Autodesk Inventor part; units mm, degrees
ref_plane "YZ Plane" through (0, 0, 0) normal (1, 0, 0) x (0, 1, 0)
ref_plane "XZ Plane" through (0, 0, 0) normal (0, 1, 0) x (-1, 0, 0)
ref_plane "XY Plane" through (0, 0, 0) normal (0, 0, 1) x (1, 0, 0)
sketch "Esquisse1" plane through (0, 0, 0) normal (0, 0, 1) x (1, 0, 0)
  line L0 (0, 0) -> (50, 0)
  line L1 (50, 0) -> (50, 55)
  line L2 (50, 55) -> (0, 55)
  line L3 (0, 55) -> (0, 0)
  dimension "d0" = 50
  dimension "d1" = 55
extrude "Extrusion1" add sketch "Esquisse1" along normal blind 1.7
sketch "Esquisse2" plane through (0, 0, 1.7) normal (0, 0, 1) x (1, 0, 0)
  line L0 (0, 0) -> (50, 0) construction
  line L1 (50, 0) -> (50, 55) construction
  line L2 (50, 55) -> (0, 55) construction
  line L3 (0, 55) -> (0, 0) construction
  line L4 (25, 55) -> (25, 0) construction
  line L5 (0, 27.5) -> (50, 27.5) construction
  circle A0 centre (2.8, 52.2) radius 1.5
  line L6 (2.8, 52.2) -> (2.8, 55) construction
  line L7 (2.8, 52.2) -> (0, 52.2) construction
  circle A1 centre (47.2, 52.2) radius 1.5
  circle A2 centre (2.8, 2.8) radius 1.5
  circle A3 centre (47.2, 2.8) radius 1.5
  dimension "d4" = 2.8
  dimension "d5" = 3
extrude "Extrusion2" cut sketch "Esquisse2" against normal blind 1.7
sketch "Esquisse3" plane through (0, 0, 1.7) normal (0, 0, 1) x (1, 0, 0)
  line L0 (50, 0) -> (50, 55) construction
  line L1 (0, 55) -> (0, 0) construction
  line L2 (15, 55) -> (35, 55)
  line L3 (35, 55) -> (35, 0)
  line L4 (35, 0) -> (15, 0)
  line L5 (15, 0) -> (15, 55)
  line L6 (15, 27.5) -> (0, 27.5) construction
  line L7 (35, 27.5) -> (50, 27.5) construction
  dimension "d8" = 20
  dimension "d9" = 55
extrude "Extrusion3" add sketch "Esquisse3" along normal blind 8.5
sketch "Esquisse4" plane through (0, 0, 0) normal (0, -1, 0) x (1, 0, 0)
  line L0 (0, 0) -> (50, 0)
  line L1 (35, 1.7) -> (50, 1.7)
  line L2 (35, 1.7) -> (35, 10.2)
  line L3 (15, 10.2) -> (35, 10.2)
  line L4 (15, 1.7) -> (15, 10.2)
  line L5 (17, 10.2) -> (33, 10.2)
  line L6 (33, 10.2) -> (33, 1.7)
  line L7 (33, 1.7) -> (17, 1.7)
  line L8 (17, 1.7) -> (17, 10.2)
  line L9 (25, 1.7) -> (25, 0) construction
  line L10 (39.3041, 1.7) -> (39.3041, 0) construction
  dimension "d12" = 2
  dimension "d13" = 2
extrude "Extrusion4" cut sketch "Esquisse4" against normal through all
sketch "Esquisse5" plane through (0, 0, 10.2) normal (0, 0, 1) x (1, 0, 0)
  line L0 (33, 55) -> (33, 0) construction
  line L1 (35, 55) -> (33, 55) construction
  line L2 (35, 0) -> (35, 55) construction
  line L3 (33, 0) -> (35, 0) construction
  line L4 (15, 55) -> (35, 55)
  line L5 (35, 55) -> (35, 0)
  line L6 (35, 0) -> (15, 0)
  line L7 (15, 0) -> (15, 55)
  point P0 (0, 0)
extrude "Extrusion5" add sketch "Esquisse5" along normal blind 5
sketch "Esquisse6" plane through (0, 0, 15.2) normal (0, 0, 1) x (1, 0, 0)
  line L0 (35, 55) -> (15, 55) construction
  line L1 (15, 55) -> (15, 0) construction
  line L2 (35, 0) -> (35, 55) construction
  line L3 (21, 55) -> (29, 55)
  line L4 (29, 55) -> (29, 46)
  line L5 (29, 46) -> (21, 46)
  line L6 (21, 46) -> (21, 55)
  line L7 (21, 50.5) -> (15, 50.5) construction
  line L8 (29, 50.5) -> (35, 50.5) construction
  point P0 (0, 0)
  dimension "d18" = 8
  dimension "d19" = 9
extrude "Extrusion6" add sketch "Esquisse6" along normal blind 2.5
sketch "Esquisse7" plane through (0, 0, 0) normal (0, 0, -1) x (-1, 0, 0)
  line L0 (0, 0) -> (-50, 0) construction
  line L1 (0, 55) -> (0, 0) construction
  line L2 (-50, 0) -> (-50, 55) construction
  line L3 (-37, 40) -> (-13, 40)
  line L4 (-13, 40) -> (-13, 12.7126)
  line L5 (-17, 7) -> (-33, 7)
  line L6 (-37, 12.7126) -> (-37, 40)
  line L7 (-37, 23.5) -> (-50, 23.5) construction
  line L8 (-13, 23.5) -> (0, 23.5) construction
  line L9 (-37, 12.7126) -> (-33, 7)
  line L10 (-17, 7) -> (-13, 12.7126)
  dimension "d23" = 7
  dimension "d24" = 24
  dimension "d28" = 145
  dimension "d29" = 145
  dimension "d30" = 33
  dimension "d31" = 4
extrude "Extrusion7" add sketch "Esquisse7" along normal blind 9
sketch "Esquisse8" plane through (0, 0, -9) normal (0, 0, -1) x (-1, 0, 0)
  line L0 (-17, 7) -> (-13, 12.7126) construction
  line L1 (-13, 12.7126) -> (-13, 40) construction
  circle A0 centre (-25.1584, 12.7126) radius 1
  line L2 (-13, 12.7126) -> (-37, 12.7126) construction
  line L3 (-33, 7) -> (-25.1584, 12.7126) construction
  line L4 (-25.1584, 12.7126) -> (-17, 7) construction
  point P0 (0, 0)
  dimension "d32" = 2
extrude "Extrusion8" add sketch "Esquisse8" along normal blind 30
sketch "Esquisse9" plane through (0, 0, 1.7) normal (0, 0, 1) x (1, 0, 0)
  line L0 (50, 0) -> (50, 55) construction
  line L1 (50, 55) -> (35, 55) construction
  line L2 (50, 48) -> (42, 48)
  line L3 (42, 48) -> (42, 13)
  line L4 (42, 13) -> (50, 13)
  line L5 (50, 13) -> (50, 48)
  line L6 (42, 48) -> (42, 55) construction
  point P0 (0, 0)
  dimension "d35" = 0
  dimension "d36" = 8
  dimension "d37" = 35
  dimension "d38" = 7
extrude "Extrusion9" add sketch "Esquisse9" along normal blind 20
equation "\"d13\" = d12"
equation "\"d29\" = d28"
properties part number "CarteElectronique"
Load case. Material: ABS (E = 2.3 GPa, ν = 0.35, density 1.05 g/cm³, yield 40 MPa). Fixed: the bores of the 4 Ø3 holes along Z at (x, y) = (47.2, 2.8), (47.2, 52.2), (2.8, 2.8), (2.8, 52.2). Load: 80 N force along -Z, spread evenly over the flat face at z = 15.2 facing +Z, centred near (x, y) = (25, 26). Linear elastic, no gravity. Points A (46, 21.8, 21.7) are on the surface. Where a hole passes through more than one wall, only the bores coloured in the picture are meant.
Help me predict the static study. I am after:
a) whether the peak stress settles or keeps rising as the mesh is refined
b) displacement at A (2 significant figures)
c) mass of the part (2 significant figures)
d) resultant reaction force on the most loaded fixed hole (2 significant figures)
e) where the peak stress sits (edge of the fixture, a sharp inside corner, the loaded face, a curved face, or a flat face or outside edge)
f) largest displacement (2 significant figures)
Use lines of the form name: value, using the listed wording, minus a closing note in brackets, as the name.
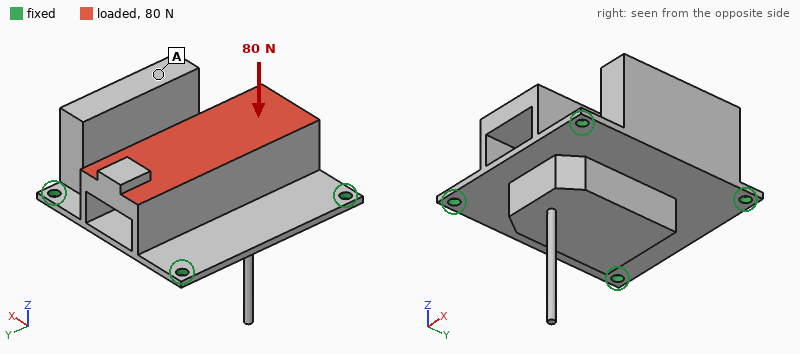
whether the peak stress settles or keeps rising as the mesh is refined: keeps rising
displacement at A: 0.36 mm
mass of the part: 26 g
resultant reaction force on the most loaded fixed hole: 23 N
where the peak stress sits: edge of the fixture
largest displacement: 0.39 mm
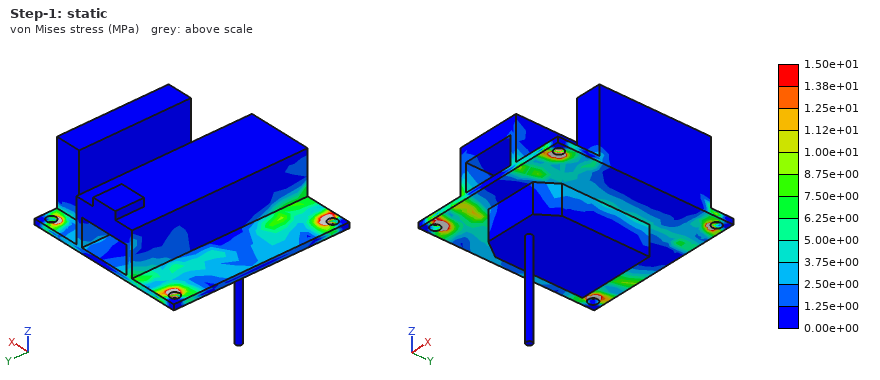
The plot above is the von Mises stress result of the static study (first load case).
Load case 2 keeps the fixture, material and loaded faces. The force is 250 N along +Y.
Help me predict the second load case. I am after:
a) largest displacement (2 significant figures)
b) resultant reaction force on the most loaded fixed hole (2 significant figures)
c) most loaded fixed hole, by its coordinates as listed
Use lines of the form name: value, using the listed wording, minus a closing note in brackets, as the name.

largest displacement: 0.76 mm
resultant reaction force on the most loaded fixed hole: 94 N
most loaded fixed hole, by its coordinates as listed: (47.2, 52.2)
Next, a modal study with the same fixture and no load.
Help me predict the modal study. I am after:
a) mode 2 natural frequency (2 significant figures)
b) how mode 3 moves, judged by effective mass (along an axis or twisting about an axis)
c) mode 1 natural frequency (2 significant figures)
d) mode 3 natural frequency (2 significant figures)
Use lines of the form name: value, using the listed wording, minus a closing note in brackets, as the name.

mode 2 natural frequency: 450 Hz
how mode 3 moves, judged by effective mass: along Z
mode 1 natural frequency: 440 Hz
mode 3 natural frequency: 550 Hz
